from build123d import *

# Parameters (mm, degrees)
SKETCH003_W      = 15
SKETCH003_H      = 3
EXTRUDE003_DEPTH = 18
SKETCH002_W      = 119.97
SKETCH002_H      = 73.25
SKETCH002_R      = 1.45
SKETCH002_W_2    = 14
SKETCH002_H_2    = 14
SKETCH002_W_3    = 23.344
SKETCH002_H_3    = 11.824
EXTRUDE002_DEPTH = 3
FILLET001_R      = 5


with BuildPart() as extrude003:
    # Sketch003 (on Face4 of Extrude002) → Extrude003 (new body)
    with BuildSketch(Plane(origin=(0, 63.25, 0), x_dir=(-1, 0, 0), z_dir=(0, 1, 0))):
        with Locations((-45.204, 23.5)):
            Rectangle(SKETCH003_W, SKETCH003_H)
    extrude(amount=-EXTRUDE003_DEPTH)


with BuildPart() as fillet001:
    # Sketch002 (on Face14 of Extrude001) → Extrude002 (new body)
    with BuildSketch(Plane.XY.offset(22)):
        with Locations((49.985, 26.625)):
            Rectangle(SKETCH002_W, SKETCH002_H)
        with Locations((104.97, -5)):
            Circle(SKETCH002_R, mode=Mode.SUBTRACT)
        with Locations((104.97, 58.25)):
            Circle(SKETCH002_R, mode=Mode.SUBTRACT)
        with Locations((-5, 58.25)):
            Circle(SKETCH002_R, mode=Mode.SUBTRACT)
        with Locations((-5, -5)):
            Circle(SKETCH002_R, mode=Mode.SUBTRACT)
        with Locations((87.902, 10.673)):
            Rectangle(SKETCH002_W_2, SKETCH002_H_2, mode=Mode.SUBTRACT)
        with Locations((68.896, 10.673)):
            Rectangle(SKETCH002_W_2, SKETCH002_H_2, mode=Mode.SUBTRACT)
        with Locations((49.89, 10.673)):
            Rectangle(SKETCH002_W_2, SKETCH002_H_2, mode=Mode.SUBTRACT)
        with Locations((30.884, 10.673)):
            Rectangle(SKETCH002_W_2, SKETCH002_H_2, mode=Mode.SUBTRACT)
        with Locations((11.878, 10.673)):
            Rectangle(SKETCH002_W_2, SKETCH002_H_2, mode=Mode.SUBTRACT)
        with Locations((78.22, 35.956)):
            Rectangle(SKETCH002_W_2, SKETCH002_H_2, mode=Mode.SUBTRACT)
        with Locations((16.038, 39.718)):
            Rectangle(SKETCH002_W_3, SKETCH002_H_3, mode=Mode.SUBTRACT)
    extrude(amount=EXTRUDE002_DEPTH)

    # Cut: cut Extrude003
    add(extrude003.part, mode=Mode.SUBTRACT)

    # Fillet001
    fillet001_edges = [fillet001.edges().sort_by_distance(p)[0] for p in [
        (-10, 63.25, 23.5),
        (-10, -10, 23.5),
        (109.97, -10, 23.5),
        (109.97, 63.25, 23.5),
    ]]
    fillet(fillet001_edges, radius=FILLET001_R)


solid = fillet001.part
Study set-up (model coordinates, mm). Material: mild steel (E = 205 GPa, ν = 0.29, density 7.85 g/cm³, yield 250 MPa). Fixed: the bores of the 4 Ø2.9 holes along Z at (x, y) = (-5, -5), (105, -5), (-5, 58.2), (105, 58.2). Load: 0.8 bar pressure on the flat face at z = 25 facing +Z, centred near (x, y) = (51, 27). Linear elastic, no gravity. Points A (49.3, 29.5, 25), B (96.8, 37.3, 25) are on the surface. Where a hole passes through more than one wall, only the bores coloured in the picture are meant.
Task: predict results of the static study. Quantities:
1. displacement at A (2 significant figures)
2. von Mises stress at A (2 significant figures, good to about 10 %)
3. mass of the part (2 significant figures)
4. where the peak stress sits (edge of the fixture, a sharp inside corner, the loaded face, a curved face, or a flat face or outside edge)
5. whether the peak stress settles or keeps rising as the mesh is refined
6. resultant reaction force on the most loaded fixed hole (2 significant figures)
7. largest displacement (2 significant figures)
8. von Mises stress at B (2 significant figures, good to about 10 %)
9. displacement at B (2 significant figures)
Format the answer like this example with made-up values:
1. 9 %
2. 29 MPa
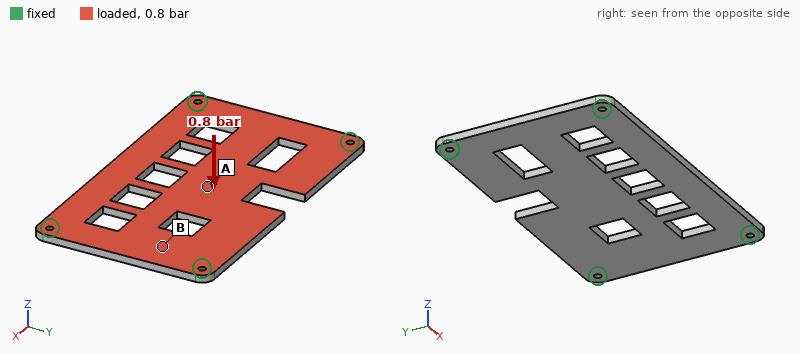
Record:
1. 0.11 mm
2. 32 MPa
3. 170 g
4. edge of the fixture
5. keeps rising
6. 150 N
7. 0.11 mm
8. 17 MPa
9. 0.026 mm
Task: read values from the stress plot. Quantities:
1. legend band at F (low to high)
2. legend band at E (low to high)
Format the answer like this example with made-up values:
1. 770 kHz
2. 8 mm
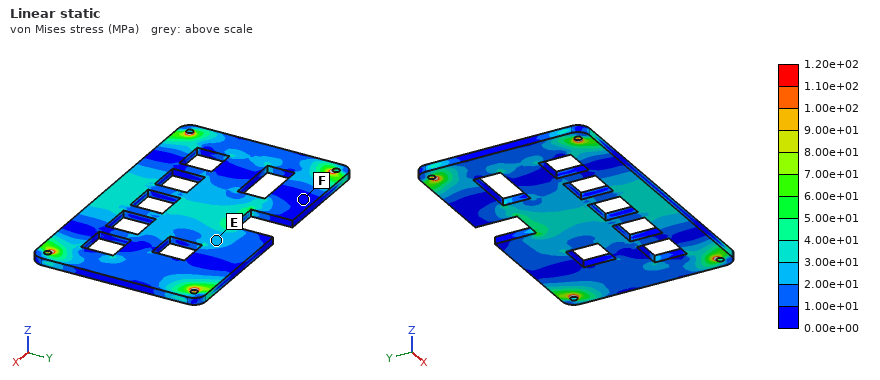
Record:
1. 0.00e+00 to 1.00e+01 MPa
2. 2.00e+01 to 3.00e+01 MPa
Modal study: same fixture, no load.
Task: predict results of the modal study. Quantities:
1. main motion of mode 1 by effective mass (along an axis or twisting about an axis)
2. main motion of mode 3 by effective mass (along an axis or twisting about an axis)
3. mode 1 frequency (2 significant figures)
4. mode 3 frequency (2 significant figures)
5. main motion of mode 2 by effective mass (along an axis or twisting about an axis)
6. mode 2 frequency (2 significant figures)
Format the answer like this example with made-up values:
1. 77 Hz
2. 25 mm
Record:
1. along Z
2. twisting about Y
3. 1000 Hz
4. 2600 Hz
5. twisting about X
6. 1700 Hz
